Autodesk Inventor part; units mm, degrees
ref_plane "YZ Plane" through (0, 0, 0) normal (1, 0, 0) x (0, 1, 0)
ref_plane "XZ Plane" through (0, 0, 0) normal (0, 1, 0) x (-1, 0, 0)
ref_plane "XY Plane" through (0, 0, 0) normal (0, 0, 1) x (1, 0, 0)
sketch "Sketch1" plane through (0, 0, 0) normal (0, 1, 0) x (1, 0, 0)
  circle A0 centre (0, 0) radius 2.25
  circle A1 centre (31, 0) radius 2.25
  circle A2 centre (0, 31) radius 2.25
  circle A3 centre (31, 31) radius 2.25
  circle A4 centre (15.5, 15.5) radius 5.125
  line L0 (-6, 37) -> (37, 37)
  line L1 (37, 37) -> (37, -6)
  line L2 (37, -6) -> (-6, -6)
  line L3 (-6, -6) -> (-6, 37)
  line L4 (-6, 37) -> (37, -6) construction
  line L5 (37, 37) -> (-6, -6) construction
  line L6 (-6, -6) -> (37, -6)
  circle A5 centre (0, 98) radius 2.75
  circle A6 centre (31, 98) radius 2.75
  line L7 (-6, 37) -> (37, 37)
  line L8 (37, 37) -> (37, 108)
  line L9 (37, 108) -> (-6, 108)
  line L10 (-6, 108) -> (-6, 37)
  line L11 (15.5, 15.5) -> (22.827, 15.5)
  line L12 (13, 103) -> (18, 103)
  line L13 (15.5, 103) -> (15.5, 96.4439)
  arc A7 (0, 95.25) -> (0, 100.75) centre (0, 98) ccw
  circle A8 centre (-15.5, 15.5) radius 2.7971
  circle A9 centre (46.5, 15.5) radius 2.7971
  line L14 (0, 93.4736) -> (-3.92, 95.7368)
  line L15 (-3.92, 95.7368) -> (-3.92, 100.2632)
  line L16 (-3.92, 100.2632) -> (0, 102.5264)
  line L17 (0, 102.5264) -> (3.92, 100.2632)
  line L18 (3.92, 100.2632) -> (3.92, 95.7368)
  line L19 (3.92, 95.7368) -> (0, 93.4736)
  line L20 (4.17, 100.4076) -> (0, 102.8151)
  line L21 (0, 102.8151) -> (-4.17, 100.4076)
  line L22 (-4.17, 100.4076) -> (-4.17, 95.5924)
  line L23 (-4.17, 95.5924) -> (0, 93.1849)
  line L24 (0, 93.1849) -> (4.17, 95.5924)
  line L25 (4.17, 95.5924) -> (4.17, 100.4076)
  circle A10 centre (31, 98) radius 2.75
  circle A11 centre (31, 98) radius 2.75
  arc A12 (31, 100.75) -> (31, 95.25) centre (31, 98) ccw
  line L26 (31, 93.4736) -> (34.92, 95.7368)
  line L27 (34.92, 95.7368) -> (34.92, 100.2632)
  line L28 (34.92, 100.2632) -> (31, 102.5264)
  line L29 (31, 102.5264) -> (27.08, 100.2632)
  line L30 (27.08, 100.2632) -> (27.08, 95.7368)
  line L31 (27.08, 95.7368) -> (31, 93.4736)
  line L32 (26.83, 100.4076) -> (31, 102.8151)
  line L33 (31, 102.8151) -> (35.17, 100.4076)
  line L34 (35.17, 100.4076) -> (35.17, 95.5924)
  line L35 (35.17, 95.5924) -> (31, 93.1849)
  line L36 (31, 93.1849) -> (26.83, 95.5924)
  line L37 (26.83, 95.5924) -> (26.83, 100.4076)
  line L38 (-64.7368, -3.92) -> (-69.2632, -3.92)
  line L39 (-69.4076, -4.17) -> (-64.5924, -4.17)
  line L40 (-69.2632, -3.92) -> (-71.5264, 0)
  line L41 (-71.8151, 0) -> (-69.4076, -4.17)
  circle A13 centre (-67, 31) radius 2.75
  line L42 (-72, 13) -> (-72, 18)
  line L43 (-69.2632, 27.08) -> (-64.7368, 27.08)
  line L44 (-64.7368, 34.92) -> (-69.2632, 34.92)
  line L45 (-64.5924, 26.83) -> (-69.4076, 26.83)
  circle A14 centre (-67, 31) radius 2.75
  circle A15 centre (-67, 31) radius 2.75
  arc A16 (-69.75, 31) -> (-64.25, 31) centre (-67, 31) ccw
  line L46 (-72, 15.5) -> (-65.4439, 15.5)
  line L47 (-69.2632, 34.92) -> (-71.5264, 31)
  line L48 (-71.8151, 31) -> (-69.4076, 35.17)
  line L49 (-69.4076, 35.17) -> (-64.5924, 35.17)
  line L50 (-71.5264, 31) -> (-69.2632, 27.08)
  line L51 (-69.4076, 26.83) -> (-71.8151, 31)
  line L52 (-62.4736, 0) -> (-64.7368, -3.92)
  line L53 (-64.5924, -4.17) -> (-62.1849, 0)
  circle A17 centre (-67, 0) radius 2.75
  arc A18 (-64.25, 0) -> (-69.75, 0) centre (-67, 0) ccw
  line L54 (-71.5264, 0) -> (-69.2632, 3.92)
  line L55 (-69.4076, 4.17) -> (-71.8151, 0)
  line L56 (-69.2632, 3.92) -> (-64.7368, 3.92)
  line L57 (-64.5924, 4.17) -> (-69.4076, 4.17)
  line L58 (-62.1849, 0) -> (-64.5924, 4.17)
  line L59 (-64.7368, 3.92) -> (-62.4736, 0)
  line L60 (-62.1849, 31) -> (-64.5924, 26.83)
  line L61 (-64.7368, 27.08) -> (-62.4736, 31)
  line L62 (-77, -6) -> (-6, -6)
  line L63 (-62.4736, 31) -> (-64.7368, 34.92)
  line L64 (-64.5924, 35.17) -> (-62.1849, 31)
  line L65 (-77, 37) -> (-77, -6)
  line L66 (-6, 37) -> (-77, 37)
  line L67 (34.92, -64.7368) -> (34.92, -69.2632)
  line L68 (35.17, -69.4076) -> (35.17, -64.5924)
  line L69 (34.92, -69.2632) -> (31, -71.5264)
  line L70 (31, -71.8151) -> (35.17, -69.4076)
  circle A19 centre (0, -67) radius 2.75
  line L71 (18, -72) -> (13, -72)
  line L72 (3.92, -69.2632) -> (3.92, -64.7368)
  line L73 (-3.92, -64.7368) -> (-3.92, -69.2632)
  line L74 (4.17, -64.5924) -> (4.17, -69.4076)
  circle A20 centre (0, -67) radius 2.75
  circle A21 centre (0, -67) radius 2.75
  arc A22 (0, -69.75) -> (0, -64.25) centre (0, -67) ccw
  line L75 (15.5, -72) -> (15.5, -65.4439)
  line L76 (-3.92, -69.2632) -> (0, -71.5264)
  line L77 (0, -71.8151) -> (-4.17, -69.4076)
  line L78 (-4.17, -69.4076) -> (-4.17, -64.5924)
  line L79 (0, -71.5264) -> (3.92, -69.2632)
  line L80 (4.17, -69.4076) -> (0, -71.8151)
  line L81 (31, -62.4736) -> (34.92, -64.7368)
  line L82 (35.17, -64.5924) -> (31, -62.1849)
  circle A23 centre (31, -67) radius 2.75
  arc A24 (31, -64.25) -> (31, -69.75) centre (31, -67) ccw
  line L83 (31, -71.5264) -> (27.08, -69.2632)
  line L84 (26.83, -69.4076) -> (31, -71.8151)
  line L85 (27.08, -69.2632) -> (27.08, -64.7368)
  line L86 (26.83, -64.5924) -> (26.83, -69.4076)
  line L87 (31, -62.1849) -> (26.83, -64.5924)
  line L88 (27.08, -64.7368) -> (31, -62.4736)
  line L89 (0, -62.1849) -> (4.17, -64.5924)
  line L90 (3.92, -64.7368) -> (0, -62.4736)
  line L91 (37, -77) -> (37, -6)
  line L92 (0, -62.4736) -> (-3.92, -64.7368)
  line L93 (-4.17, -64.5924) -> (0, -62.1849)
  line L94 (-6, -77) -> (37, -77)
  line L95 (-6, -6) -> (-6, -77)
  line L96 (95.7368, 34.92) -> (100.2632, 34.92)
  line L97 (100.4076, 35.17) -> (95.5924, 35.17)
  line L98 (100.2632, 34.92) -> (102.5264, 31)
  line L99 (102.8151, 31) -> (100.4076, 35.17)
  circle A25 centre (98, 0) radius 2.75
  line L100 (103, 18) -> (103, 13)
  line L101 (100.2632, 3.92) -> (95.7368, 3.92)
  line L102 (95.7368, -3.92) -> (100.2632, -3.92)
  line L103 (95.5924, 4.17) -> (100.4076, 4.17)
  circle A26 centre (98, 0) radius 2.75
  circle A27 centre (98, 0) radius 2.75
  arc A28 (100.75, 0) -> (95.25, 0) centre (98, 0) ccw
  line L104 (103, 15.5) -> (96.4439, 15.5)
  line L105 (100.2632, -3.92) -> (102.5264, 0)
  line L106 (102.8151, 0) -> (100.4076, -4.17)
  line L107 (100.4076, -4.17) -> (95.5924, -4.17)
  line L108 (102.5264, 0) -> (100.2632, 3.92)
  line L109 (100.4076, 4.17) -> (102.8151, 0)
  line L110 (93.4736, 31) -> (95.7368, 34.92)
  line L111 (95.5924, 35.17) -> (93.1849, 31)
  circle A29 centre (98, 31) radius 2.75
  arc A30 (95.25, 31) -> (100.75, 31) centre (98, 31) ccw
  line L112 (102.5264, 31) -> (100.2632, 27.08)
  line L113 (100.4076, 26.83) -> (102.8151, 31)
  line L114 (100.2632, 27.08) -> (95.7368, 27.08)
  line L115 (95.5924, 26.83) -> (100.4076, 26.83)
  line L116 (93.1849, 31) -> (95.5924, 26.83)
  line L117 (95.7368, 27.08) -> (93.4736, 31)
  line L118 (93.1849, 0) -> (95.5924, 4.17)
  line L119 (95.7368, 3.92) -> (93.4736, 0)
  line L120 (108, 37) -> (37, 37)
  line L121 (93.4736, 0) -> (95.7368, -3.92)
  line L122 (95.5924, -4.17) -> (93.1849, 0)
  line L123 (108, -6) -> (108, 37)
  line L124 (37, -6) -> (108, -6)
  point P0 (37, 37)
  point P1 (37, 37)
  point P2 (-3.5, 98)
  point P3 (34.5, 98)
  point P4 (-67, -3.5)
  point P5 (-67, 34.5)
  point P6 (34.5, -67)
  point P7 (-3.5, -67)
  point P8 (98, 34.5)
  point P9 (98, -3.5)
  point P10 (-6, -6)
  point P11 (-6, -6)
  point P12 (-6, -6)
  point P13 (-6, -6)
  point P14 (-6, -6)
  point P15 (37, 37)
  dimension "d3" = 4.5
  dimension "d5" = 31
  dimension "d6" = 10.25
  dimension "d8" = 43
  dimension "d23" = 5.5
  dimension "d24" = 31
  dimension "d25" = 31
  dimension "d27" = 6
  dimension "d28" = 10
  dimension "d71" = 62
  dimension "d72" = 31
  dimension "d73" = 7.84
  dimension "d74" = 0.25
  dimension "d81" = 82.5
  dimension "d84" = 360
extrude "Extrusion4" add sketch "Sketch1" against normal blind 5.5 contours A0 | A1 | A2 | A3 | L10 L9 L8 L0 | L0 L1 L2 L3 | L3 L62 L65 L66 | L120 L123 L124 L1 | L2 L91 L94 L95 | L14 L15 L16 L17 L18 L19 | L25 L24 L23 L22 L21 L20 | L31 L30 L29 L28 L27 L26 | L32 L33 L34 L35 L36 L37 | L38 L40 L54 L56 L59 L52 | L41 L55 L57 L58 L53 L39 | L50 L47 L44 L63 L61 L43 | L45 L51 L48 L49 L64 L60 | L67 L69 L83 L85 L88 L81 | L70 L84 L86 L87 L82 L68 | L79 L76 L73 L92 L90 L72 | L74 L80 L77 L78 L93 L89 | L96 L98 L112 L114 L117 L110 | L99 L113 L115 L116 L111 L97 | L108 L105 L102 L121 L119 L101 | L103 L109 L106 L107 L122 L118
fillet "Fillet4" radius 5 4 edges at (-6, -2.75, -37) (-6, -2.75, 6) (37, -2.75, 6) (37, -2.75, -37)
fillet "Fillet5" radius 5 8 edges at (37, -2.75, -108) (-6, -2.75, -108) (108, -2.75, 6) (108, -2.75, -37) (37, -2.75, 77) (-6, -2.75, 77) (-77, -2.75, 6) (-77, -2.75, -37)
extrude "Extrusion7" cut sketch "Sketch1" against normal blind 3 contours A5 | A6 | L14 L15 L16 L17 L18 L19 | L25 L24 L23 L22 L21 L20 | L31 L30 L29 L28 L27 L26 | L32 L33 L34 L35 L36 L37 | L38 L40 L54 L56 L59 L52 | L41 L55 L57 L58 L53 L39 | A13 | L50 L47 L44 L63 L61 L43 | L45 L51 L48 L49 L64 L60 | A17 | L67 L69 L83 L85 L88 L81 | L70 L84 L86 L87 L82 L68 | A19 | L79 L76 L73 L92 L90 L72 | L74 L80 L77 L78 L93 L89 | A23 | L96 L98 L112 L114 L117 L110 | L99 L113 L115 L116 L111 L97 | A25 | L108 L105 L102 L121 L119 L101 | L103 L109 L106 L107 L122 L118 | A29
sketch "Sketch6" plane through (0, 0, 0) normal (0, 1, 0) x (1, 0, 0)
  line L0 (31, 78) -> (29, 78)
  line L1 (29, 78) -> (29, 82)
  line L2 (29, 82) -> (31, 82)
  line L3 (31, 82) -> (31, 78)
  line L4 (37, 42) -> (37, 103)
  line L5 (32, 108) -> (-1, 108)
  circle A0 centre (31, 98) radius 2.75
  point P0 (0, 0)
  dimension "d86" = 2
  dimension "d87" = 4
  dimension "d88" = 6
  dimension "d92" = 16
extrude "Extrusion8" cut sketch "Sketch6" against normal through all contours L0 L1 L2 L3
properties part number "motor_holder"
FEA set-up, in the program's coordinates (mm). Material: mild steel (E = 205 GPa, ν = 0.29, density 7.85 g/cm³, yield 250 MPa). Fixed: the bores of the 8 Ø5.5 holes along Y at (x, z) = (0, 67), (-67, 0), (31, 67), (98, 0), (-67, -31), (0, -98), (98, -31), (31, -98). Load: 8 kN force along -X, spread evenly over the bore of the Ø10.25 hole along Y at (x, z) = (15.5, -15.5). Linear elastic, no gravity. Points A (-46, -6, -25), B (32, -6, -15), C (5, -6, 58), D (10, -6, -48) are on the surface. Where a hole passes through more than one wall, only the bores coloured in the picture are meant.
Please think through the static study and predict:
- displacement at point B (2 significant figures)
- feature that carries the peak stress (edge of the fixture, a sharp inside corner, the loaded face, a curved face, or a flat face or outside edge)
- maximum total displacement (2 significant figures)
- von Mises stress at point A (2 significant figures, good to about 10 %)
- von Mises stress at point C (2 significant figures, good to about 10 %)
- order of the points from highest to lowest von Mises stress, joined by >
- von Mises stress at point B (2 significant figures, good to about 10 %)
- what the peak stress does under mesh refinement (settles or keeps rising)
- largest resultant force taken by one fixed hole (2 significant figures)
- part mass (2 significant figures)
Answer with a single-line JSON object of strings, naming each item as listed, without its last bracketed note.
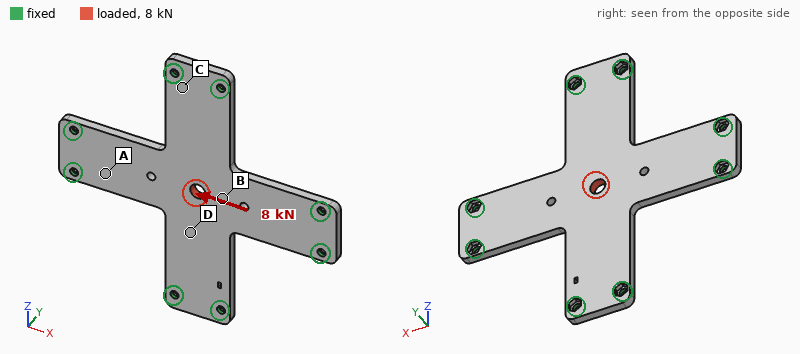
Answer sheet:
{"displacement at point B": "7.7 µm", "feature that carries the peak stress": "edge of the fixture", "maximum total displacement": "9.4 µm", "von Mises stress at point A": "20 MPa", "von Mises stress at point C": "12 MPa", "order of the points from highest to lowest von Mises stress, joined by >": "B > A > C > D", "von Mises stress at point B": "30 MPa", "what the peak stress does under mesh refinement": "keeps rising", "largest resultant force taken by one fixed hole": "1.8 kN", "part mass": "590 g"}
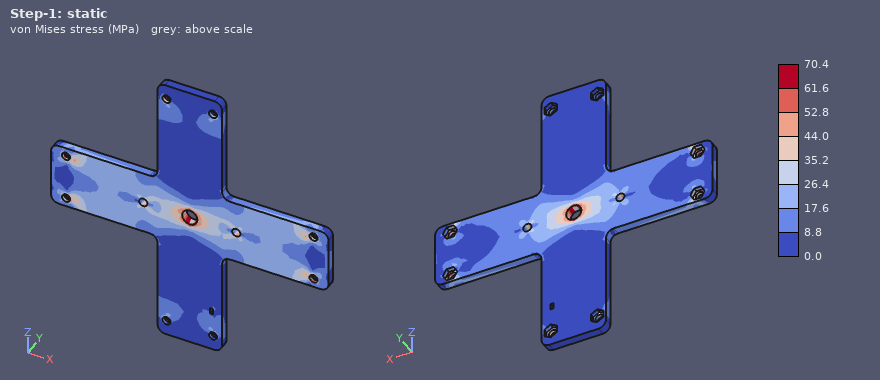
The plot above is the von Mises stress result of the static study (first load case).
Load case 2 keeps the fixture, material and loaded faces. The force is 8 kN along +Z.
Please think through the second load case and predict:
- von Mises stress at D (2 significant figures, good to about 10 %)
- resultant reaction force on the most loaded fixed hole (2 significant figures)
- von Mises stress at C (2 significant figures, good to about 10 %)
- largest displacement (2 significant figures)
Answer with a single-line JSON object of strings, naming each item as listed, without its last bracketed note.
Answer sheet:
{"von Mises stress at D": "21 MPa", "resultant reaction force on the most loaded fixed hole": "1.8 kN", "von Mises stress at C": "24 MPa", "largest displacement": "9.2 µm"}
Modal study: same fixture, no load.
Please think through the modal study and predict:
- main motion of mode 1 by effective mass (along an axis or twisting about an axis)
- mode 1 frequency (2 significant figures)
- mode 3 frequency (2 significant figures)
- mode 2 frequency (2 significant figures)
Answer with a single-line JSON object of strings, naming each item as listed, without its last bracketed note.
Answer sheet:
{"main motion of mode 1 by effective mass": "along Y", "mode 1 frequency": "1200 Hz", "mode 3 frequency": "2700 Hz", "mode 2 frequency": "2700 Hz"}
